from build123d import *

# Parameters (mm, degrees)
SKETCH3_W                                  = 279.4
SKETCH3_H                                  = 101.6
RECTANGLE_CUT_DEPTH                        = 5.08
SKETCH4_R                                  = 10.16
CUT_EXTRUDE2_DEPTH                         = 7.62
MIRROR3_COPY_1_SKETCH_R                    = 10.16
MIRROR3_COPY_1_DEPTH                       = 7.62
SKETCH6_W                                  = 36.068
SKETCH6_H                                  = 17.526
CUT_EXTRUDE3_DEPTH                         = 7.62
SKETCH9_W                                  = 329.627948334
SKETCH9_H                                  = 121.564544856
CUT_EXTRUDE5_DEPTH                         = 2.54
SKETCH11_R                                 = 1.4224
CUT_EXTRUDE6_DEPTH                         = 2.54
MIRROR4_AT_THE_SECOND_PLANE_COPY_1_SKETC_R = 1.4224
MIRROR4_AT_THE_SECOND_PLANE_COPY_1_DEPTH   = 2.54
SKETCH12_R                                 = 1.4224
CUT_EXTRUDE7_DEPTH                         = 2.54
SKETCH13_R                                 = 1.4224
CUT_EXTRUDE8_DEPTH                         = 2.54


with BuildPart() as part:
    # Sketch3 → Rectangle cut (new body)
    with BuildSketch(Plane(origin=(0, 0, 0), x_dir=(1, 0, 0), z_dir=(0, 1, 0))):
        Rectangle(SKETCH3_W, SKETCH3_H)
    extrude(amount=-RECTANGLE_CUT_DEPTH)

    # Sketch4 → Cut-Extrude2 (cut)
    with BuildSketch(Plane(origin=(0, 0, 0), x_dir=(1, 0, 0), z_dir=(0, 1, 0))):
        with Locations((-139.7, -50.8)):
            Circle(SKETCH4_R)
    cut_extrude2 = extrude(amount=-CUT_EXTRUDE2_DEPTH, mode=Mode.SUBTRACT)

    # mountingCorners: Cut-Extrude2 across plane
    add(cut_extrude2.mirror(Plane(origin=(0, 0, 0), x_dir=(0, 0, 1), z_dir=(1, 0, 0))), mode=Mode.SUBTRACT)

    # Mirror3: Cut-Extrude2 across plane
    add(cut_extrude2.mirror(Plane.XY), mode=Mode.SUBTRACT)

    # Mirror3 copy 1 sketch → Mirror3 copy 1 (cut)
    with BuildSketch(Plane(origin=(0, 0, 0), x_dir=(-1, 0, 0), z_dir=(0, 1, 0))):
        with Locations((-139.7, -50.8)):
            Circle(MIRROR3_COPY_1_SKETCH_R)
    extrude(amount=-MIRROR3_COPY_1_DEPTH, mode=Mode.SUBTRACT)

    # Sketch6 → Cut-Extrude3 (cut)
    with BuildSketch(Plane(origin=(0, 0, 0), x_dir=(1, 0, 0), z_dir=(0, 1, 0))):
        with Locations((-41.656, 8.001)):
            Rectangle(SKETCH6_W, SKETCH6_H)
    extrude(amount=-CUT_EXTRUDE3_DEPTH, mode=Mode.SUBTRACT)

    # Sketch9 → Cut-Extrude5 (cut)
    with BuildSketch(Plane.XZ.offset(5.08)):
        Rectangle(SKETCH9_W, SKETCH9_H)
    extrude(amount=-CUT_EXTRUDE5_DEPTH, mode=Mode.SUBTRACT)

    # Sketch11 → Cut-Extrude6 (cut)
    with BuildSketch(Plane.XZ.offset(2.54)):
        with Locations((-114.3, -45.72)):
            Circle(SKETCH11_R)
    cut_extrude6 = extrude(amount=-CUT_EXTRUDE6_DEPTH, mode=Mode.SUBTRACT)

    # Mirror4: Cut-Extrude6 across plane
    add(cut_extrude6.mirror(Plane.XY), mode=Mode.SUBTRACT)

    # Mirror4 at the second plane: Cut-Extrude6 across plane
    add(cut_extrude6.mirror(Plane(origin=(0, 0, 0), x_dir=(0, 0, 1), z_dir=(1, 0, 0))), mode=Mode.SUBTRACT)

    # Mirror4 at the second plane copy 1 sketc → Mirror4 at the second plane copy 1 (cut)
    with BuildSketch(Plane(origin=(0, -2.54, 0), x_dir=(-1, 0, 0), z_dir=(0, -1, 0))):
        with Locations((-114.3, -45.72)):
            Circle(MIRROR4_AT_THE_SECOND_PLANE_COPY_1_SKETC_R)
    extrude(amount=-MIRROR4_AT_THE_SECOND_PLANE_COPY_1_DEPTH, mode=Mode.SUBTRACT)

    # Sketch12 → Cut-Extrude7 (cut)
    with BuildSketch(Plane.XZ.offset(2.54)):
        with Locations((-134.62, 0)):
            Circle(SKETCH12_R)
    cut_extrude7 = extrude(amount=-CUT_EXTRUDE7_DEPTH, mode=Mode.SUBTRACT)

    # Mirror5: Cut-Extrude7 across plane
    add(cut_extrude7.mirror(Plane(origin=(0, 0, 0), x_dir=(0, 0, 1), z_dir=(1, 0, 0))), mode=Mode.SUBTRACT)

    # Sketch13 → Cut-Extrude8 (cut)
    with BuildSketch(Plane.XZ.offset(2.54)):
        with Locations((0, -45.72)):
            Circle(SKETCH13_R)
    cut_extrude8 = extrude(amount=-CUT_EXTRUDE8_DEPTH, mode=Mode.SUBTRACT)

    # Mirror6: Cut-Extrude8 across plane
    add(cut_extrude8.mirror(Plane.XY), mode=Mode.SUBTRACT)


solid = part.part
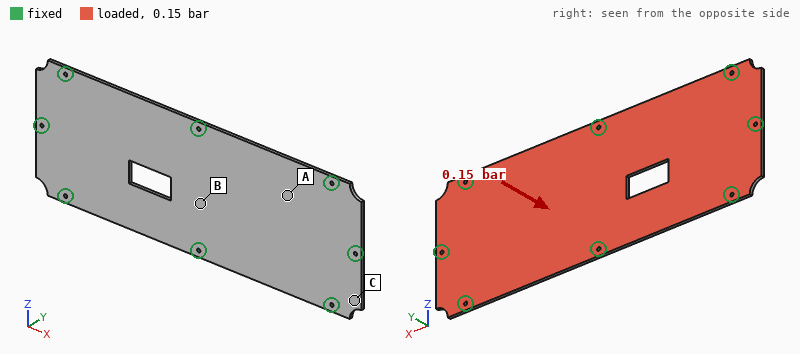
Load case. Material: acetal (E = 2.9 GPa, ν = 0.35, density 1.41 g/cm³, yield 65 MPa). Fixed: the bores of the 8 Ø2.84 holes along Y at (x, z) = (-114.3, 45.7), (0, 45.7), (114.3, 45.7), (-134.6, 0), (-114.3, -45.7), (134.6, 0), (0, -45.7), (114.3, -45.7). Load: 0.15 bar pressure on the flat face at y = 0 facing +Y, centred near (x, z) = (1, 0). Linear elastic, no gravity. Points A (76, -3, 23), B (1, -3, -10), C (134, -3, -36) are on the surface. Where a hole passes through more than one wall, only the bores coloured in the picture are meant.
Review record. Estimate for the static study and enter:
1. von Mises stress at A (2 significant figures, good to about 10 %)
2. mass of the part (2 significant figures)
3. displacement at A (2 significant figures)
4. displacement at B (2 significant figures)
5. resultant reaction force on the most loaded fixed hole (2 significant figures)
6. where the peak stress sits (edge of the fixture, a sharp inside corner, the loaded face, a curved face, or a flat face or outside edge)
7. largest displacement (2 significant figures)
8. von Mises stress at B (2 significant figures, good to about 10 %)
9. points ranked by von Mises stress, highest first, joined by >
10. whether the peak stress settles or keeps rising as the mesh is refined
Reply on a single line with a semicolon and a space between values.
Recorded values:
6.5 MPa; 98 g; 2.3 mm; 1.7 mm; 89 N; edge of the fixture; 3.2 mm; 11 MPa; B > A > C; keeps rising
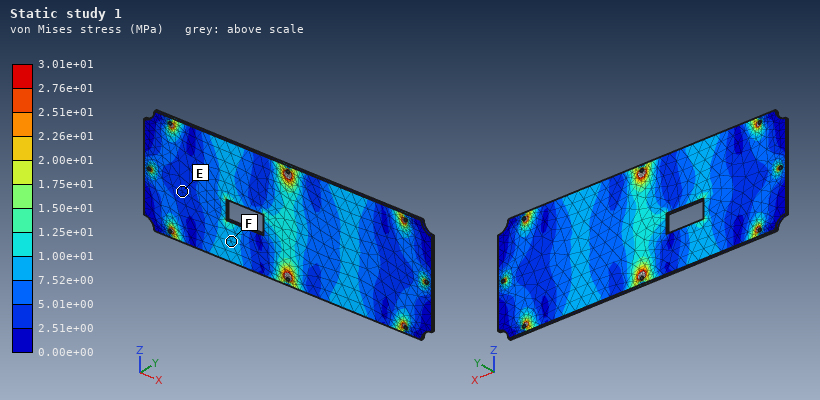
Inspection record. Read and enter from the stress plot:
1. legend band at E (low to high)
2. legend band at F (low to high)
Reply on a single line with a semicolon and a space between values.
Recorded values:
2.51e+00 to 5.01e+00 MPa; 7.52e+00 to 1.00e+01 MPa
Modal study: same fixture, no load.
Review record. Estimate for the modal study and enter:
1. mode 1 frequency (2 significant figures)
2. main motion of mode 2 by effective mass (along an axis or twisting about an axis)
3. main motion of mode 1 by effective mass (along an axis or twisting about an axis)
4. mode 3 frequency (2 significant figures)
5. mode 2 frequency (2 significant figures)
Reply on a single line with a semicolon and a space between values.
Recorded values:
210 Hz; along Y; twisting about Z; 330 Hz; 230 Hz
